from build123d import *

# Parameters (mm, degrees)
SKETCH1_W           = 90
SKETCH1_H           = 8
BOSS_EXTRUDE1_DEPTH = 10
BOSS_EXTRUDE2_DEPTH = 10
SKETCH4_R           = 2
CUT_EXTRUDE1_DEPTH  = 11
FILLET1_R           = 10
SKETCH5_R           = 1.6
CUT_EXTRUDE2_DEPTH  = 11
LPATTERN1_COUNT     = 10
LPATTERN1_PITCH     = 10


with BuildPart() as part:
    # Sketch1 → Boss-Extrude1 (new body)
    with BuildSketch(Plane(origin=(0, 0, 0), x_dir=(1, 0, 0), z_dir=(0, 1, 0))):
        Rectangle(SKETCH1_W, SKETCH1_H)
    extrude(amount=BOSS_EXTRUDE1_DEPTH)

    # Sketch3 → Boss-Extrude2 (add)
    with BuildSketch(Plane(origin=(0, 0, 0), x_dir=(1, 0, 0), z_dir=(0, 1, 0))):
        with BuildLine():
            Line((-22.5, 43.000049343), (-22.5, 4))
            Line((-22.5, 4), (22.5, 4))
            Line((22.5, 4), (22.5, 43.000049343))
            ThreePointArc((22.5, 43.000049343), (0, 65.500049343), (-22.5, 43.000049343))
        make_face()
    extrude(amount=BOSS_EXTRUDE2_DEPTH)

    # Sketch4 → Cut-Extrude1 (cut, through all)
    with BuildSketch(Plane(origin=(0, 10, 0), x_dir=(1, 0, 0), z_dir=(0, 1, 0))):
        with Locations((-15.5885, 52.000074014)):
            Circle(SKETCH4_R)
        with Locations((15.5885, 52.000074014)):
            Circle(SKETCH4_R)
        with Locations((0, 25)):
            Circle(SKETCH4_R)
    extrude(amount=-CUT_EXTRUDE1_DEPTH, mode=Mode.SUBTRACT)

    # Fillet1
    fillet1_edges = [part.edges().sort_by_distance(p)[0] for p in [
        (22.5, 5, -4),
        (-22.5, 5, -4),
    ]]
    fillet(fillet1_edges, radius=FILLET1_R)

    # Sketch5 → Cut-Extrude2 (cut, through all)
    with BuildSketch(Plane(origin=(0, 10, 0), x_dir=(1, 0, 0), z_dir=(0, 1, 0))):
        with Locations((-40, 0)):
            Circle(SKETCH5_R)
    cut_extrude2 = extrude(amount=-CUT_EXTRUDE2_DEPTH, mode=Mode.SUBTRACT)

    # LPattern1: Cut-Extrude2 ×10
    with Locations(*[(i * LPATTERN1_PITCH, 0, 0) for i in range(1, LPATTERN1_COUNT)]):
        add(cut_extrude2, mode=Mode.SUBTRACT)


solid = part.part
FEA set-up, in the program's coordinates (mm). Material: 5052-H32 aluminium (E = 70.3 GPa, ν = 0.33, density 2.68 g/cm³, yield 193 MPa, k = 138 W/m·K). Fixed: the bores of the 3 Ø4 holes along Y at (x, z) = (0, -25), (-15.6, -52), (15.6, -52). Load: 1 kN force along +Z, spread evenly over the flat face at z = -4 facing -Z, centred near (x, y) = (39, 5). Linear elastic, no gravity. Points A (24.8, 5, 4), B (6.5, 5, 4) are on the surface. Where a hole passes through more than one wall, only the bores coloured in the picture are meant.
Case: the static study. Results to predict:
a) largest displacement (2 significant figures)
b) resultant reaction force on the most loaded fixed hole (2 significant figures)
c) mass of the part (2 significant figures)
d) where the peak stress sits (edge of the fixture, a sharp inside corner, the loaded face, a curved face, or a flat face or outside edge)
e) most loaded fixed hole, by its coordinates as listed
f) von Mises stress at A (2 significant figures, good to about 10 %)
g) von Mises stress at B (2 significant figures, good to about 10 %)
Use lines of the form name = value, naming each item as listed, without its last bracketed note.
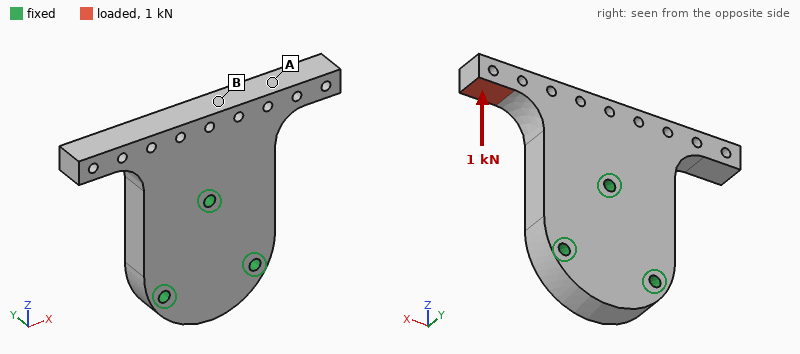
largest displacement = 0.11 mm
resultant reaction force on the most loaded fixed hole = 950 N
mass of the part = 86 g
where the peak stress sits = a curved face
most loaded fixed hole, by its coordinates as listed = (15.6, -52)
von Mises stress at A = 86 MPa
von Mises stress at B = 20 MPa
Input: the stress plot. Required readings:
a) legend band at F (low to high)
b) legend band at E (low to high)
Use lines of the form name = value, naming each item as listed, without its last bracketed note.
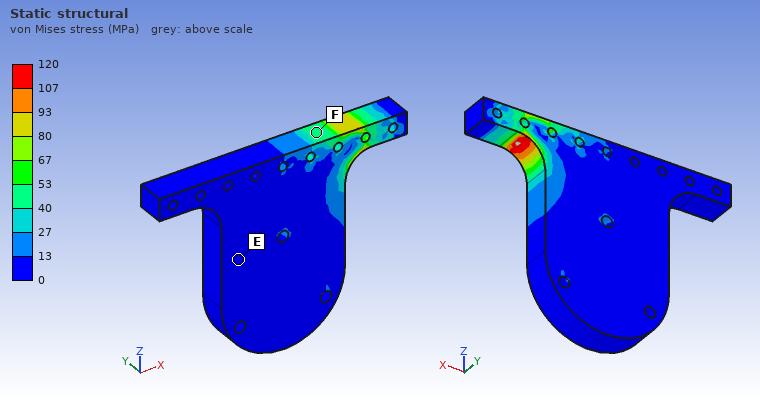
legend band at F = 40 to 53 MPa
legend band at E = 0 to 13 MPa
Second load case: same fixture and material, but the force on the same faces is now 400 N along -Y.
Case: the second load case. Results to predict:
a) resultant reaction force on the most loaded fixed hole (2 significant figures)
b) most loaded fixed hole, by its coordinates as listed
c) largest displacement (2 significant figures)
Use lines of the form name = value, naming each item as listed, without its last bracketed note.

resultant reaction force on the most loaded fixed hole = 530 N
most loaded fixed hole, by its coordinates as listed = (0, -25)
largest displacement = 0.13 mm
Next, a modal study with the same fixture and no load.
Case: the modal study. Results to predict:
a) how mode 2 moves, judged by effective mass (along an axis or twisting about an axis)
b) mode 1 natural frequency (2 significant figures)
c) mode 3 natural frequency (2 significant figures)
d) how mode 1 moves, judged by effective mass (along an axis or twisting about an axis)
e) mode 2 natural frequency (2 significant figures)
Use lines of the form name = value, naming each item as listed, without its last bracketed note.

how mode 2 moves, judged by effective mass = along Y
mode 1 natural frequency = 4400 Hz
mode 3 natural frequency = 8700 Hz
how mode 1 moves, judged by effective mass = twisting about Z
mode 2 natural frequency = 5000 Hz
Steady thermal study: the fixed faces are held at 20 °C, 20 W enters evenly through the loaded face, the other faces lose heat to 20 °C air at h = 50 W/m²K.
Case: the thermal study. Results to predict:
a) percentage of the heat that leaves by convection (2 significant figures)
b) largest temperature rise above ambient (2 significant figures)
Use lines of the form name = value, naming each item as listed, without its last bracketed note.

percentage of the heat that leaves by convection = 16 %
largest temperature rise above ambient = 52 K
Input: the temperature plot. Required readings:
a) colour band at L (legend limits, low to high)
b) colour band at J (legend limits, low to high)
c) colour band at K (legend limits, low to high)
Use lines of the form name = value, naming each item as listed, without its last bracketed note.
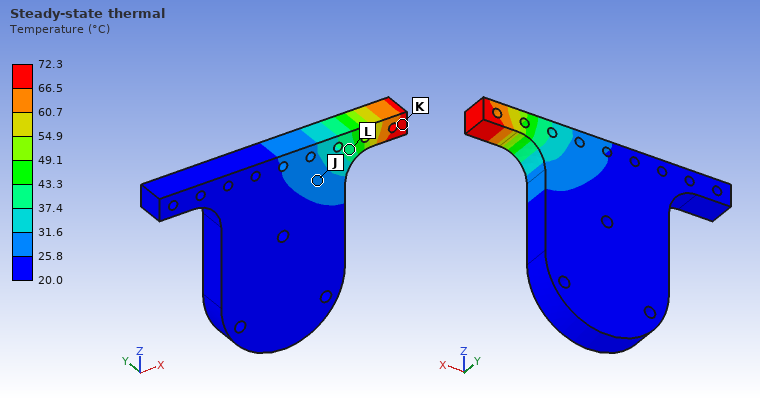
colour band at L = 37.4 to 43.3 °C
colour band at J = 25.8 to 31.6 °C
colour band at K = 66.5 to 72.3 °C
